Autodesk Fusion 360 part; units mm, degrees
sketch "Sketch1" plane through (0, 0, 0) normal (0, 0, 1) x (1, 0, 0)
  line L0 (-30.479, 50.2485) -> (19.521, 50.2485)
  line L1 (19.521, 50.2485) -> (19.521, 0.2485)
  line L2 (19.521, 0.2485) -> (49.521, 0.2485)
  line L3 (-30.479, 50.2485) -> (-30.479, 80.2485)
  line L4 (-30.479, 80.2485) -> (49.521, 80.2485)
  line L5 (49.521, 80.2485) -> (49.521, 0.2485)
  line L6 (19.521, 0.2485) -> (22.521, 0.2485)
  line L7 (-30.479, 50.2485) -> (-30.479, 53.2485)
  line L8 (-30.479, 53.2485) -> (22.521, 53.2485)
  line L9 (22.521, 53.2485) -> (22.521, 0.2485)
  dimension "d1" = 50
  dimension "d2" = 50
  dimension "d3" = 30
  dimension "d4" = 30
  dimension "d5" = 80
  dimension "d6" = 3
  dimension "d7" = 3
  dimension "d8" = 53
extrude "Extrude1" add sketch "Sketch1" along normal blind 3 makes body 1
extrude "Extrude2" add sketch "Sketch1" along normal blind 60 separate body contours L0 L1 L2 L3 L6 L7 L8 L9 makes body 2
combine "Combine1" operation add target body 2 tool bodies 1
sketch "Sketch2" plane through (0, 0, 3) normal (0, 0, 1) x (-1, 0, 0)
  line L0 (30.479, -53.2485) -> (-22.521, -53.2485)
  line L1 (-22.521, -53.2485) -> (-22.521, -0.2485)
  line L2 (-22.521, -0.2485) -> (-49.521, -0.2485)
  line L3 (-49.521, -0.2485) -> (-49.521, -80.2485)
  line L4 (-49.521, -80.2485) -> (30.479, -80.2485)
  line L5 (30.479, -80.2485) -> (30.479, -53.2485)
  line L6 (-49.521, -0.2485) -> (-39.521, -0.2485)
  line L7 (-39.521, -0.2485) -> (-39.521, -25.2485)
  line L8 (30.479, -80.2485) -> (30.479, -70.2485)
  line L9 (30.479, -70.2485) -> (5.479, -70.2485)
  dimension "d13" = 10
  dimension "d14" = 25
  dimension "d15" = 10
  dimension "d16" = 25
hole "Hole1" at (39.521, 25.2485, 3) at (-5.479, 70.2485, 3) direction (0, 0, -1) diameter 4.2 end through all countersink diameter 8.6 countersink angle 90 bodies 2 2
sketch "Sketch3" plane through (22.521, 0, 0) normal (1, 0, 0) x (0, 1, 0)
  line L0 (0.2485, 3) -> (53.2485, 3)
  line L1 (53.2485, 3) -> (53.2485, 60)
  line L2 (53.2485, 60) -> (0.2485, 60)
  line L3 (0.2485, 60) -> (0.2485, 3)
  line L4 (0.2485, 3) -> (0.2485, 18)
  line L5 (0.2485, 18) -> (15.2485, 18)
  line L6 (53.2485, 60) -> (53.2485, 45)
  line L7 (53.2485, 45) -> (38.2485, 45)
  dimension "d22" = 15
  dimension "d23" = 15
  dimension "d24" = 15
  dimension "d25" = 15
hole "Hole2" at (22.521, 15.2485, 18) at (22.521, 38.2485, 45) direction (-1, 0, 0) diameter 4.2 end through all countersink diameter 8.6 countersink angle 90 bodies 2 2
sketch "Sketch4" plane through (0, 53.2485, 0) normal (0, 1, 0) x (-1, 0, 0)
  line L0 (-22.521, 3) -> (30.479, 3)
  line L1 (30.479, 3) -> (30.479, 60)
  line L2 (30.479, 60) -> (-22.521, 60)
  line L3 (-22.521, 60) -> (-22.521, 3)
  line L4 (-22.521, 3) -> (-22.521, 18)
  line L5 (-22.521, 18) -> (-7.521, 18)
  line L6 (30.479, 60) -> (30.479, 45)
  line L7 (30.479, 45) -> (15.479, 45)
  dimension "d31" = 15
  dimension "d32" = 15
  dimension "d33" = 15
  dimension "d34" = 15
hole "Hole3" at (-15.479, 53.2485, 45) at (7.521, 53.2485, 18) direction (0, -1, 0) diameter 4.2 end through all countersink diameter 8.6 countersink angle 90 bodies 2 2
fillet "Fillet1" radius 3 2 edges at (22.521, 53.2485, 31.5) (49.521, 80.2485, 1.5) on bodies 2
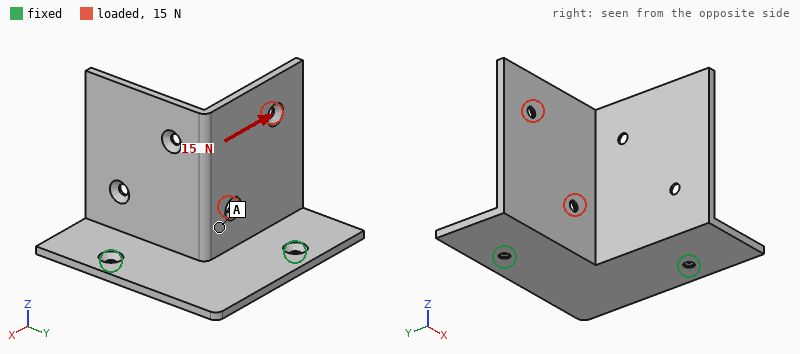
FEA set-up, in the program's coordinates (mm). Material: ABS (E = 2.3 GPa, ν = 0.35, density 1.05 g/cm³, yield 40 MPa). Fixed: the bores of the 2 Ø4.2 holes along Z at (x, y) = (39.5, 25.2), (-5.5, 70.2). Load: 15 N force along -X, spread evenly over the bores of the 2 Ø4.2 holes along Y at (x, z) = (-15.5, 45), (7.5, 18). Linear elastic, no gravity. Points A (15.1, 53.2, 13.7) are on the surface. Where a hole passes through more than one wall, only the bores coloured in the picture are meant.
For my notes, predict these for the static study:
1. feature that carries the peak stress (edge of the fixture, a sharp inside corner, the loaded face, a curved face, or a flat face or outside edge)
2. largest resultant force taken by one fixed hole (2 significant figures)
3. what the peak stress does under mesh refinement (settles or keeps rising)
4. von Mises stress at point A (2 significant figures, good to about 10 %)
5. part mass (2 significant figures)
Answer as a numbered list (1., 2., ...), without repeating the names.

1. edge of the fixture
2. 9.9 N
3. keeps rising
4. 0.82 MPa
5. 30 g
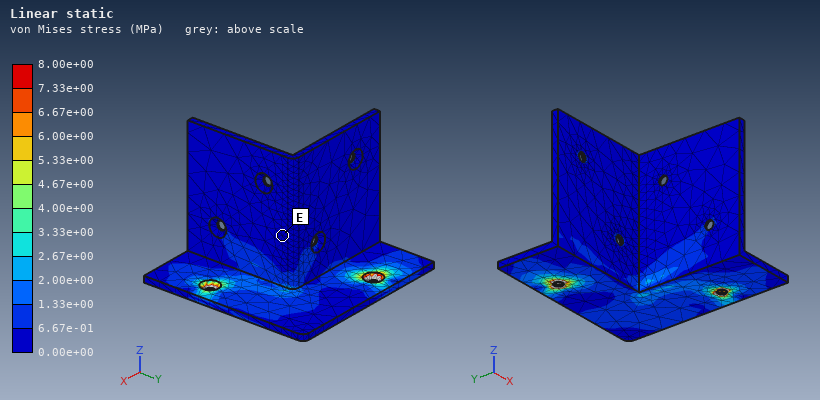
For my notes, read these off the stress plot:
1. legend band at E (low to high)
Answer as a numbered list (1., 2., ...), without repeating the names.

1. 0.00e+00 to 6.67e-01 MPa
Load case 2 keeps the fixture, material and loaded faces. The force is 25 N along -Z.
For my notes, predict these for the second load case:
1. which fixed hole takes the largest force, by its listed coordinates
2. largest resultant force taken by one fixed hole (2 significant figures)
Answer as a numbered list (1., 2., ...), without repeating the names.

1. (-5.5, 70.2)
2. 23 N
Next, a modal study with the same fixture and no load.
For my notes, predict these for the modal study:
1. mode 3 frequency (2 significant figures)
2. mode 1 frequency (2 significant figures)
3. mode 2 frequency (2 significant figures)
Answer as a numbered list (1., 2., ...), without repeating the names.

1. 350 Hz
2. 120 Hz
3. 310 Hz
